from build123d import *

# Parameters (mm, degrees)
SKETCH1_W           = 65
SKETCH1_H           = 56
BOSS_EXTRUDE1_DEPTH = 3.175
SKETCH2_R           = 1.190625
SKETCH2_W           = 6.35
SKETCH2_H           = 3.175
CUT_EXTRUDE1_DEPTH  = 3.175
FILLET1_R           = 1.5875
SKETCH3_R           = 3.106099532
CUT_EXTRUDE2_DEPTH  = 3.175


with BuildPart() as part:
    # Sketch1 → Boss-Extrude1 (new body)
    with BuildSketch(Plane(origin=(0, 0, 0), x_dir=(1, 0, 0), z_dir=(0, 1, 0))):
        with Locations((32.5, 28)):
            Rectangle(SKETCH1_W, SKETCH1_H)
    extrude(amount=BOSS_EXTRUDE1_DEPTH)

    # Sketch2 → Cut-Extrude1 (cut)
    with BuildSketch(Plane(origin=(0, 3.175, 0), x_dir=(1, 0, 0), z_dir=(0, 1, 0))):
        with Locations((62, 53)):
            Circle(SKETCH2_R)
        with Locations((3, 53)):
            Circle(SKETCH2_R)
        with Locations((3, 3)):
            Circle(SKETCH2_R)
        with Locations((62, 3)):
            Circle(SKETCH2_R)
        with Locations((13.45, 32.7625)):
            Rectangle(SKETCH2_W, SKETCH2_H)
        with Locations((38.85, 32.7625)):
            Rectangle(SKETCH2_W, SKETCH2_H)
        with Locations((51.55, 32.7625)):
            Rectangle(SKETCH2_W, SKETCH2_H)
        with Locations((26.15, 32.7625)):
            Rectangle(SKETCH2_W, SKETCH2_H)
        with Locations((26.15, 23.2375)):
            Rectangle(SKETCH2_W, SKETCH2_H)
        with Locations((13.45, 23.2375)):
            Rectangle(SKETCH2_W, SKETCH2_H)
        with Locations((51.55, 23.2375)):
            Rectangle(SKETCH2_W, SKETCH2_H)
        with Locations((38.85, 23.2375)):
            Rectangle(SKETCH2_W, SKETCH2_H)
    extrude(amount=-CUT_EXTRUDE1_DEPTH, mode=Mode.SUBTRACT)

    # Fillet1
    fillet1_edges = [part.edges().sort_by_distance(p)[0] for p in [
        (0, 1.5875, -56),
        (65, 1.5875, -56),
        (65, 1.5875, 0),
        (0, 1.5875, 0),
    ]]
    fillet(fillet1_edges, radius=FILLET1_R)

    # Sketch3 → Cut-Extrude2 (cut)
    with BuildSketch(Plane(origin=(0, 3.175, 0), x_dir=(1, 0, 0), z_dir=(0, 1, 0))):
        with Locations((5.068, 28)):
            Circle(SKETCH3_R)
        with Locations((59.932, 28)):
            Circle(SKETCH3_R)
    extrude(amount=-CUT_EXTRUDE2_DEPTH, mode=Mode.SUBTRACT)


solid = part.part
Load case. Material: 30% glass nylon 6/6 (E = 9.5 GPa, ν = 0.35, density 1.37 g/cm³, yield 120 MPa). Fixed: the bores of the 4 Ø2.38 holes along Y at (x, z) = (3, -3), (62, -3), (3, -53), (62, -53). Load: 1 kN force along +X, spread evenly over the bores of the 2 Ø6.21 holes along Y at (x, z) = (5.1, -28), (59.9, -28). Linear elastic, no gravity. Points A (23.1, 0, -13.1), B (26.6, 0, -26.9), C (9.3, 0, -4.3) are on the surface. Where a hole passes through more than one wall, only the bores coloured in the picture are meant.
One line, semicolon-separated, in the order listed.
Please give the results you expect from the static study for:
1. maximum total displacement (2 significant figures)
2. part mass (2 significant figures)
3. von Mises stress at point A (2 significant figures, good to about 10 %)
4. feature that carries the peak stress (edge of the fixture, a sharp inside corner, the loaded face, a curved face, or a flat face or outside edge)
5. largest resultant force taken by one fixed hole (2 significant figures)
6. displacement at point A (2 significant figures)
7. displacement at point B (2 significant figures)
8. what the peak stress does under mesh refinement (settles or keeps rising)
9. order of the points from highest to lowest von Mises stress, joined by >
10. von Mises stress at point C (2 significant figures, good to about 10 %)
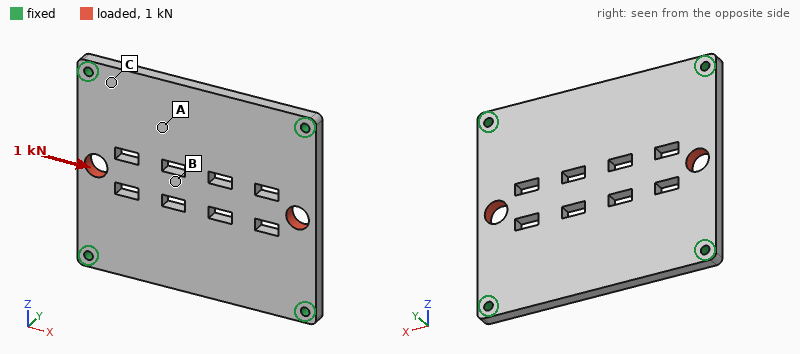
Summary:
54 µm; 15 g; 4.7 MPa; edge of the fixture; 270 N; 18 µm; 25 µm; keeps rising; C > A > B; 8.5 MPa
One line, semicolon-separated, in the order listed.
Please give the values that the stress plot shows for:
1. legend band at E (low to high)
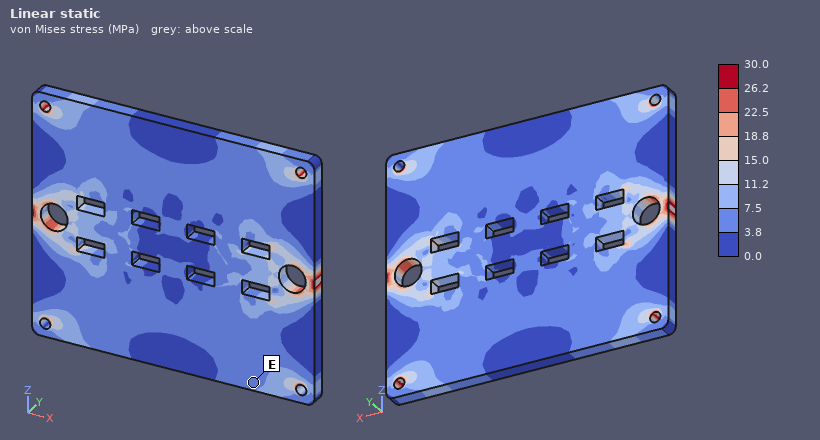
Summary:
3.8 to 7.5 MPa
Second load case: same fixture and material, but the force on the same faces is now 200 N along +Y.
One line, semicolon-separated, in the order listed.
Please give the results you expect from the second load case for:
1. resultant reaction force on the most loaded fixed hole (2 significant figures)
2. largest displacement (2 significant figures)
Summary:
50 N; 0.26 mm
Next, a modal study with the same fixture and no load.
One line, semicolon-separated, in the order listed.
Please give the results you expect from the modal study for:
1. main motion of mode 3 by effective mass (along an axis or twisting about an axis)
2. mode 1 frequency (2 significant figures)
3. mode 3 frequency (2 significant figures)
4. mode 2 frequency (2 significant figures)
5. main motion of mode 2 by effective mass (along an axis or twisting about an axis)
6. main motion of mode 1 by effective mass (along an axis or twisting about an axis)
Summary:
twisting about Z; 1600 Hz; 3300 Hz; 2700 Hz; twisting about X; along Y
